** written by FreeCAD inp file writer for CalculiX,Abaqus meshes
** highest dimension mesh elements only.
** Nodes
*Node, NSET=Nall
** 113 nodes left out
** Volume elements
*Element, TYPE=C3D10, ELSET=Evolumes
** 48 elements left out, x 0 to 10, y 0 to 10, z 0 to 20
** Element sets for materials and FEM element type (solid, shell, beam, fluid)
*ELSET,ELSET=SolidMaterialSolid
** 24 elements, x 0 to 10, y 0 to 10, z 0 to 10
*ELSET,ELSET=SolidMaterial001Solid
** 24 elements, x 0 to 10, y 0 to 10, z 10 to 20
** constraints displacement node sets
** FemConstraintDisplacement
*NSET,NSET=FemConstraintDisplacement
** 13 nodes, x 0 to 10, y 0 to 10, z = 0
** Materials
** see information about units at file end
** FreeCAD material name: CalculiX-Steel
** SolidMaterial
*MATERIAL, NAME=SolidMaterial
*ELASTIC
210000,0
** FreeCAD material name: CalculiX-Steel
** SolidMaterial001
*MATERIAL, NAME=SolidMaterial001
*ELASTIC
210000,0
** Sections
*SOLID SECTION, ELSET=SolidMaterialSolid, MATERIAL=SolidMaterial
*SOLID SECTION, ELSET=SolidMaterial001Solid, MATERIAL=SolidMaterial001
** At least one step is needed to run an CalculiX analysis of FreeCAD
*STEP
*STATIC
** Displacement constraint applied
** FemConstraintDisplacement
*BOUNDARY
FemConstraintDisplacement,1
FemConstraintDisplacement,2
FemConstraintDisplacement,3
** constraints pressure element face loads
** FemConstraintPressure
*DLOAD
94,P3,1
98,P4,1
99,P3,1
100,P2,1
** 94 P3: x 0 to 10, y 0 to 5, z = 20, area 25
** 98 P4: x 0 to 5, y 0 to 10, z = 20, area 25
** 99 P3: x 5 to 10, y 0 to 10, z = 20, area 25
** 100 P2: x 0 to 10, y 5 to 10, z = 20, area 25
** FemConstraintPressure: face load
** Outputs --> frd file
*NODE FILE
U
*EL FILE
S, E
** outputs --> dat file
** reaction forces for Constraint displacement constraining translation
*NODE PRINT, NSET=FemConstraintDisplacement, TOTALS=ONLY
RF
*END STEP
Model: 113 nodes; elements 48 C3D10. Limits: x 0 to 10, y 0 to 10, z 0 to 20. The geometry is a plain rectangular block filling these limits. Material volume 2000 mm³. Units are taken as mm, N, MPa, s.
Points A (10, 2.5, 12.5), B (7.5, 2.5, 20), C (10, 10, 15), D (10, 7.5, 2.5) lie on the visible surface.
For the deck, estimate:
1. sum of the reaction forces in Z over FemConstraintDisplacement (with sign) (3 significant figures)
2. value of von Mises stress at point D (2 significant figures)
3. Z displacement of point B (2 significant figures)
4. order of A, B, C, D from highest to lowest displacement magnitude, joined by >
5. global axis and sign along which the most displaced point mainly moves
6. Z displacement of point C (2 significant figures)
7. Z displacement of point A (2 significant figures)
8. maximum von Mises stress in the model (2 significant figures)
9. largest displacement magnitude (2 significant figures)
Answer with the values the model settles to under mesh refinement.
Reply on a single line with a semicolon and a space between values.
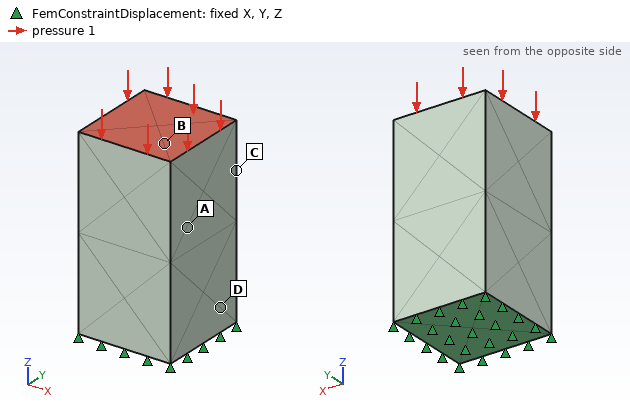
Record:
100 N; 1.0 MPa; -9.5e-05 mm; B > C > A > D; -Z; -7.1e-05 mm; -6.0e-05 mm; 1.0 MPa; 9.5e-05 mm
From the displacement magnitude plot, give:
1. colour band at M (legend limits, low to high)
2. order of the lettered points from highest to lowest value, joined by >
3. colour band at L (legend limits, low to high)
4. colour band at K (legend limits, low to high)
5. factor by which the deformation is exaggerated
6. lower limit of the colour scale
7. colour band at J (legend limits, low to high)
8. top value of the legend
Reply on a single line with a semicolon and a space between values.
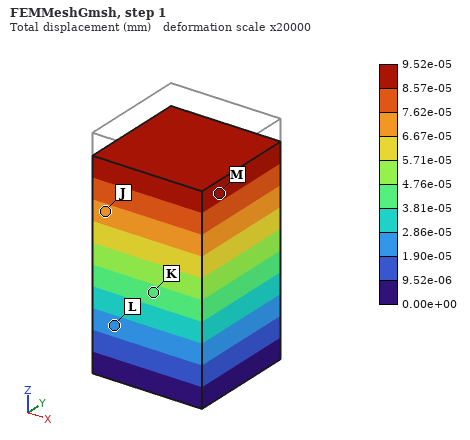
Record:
8.57e-05 to 9.52e-05 mm; M > J > K > L; 1.90e-05 to 2.86e-05 mm; 3.81e-05 to 4.76e-05 mm; 20000; 0.00e+00 mm; 6.67e-05 to 7.62e-05 mm; 9.52e-05 mm
